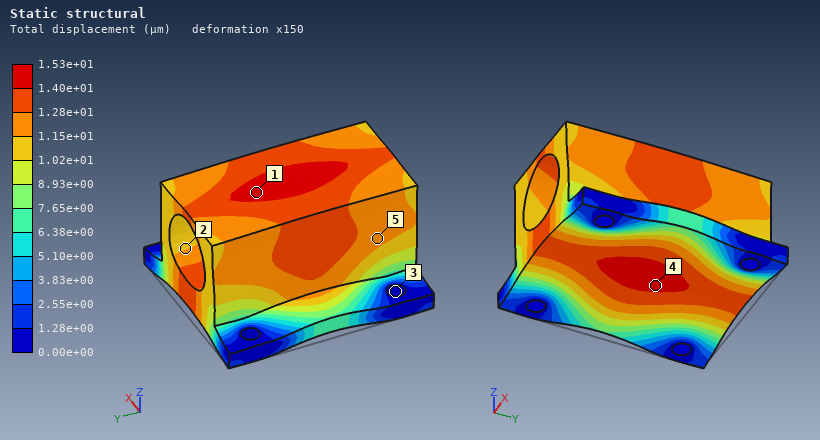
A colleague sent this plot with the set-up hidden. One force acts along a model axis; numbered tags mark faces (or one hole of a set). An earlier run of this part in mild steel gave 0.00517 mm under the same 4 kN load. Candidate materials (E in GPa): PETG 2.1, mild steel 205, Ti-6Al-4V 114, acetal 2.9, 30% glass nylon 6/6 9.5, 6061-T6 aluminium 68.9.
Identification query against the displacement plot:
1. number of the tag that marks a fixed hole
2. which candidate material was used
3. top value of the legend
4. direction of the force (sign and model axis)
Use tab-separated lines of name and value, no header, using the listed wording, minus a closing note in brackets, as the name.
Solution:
number of the tag that marks a fixed hole	3
which candidate material was used	6061-T6 aluminium
top value of the legend	1.53e+01 µm
direction of the force	+Z
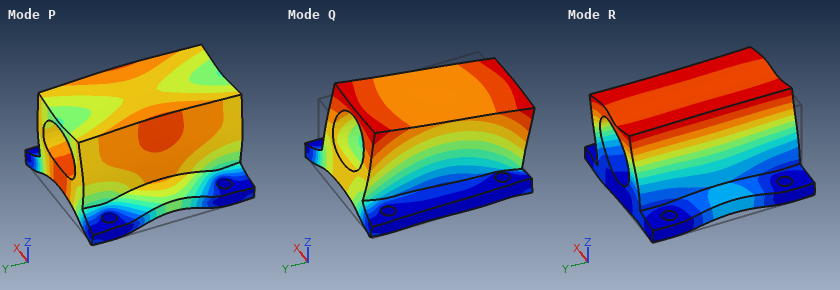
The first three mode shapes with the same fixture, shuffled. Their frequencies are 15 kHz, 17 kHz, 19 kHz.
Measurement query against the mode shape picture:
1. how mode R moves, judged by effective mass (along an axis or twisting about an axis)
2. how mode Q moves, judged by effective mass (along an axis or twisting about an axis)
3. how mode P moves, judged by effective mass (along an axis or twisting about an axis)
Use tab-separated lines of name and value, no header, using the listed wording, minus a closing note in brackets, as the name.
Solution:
how mode R moves, judged by effective mass	along X
how mode Q moves, judged by effective mass	along Y
how mode P moves, judged by effective mass	along Z
